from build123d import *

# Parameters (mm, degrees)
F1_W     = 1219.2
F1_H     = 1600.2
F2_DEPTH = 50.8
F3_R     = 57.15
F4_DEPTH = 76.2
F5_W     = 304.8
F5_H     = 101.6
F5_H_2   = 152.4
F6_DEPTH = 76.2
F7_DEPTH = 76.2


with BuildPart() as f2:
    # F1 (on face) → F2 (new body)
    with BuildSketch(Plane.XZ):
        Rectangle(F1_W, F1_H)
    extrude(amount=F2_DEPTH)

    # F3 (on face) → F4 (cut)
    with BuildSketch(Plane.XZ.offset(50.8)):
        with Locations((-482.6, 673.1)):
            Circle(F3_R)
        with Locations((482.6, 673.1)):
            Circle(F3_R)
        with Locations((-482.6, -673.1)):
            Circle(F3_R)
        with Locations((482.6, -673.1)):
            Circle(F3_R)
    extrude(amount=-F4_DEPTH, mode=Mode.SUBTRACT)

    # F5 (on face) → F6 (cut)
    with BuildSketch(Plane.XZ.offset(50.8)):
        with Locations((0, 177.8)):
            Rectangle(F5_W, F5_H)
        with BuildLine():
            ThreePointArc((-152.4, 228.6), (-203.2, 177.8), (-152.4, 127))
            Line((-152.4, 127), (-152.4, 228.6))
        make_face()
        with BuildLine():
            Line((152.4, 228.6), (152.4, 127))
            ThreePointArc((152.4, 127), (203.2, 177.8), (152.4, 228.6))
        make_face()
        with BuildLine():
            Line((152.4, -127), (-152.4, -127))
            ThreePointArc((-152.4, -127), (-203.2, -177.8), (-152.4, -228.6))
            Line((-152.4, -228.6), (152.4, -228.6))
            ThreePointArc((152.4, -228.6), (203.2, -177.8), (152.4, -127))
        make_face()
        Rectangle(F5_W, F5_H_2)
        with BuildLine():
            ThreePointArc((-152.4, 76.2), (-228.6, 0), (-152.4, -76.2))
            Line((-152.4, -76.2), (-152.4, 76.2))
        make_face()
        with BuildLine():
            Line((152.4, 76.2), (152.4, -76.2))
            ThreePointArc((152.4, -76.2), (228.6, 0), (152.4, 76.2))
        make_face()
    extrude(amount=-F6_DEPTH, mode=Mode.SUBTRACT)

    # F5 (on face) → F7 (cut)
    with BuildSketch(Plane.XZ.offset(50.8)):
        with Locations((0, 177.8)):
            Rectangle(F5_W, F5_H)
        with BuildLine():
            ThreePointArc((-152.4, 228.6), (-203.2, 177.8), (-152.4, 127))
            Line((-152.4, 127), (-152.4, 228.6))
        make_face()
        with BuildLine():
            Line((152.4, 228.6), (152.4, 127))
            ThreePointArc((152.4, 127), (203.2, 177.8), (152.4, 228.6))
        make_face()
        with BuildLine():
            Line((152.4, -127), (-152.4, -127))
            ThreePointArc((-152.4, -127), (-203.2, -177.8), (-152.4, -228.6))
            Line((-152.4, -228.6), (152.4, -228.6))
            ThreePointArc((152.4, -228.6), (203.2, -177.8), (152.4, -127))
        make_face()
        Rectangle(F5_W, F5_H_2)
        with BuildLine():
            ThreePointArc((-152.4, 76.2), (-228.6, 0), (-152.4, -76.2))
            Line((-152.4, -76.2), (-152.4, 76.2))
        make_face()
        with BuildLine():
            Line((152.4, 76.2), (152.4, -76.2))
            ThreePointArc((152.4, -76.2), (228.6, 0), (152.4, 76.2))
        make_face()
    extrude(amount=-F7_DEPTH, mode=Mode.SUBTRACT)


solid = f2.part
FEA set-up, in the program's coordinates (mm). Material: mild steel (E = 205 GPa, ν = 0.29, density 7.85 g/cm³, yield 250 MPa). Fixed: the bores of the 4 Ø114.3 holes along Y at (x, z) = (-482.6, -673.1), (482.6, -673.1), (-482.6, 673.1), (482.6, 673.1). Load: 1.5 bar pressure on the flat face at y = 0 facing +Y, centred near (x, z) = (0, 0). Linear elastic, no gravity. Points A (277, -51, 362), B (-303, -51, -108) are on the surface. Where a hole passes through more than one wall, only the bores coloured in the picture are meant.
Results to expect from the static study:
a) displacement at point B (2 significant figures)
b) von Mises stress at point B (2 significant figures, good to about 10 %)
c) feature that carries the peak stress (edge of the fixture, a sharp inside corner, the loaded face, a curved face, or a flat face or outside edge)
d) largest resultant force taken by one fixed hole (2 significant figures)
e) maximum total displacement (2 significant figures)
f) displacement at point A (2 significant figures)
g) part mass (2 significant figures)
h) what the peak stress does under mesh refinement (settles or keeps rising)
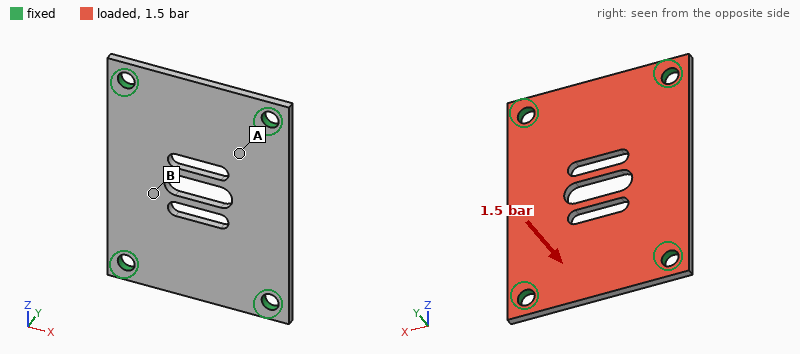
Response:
0.67 mm
25 MPa
edge of the fixture
66 kN
0.84 mm
0.41 mm
700 kg
keeps rising
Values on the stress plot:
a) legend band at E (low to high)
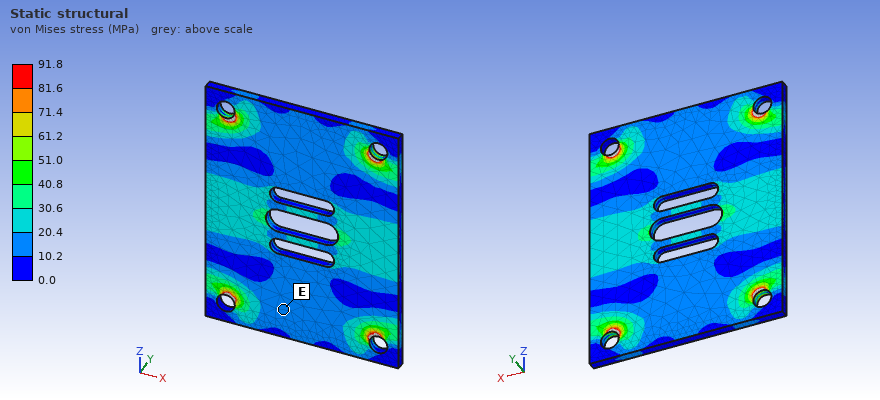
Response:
10.2 to 20.4 MPa
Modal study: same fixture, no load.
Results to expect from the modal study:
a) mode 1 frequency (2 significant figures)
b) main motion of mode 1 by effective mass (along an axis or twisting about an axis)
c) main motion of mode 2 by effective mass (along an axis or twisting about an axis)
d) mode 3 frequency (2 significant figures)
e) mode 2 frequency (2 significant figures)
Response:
140 Hz
along Y
twisting about Z
270 Hz
190 Hz
